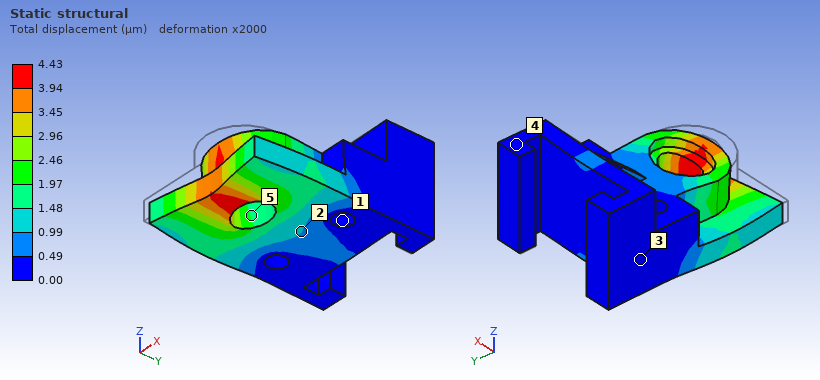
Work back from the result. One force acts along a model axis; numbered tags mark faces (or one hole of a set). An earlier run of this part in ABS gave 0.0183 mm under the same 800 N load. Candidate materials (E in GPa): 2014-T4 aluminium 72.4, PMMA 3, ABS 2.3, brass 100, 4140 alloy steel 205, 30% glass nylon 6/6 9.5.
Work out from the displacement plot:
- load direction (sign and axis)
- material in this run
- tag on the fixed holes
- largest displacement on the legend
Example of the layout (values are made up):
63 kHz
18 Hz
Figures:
+Y
30% glass nylon 6/6
1
4.43 µm
